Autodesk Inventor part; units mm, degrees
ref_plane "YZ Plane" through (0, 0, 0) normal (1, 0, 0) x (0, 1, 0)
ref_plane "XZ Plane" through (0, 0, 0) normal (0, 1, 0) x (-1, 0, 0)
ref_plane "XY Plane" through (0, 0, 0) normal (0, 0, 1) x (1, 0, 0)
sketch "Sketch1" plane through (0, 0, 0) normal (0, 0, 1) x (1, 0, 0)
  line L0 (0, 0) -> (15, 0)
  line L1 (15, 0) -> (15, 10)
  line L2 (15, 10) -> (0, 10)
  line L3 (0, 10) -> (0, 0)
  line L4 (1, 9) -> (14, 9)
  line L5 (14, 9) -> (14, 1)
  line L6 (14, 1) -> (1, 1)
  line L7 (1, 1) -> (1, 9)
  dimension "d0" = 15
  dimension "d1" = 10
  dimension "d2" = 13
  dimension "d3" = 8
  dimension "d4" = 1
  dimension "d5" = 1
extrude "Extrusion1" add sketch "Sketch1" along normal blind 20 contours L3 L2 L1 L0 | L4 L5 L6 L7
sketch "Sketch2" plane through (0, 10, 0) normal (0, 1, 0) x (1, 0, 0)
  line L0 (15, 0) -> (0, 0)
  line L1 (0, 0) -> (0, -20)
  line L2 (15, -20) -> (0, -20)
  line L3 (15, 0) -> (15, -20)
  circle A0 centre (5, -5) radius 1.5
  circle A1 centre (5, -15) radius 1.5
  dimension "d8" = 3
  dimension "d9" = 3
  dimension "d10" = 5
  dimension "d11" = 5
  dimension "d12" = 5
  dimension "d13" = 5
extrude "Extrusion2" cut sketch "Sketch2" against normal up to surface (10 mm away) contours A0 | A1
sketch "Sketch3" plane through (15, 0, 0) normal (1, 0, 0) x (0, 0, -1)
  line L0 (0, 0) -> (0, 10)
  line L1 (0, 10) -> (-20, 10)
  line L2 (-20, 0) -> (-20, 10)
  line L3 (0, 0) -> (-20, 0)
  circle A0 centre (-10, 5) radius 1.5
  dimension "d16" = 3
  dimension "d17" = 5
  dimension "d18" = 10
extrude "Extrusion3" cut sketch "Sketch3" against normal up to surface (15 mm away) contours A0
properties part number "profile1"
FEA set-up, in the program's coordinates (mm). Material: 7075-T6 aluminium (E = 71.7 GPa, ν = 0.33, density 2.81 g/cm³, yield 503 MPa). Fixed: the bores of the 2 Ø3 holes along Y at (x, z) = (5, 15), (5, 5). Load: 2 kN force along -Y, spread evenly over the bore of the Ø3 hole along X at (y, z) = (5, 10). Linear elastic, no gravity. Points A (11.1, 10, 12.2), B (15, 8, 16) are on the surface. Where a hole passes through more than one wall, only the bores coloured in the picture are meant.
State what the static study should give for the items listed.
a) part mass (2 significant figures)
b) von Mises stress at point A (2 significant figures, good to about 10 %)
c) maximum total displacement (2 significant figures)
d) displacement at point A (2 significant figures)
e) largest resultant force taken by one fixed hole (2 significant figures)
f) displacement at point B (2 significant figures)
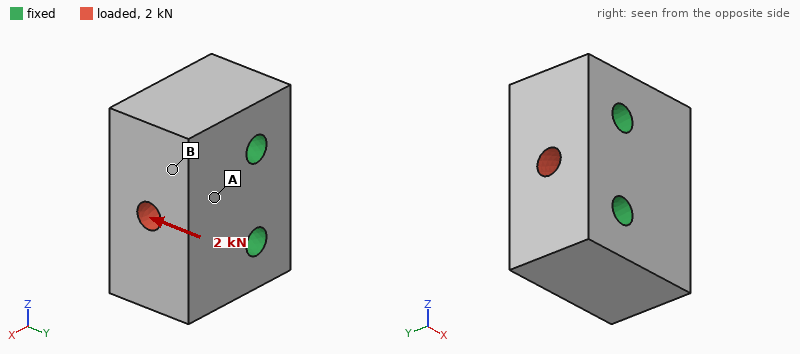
7.7 g
11 MPa
4.4 µm
2.8 µm
1.0 kN
2.7 µm
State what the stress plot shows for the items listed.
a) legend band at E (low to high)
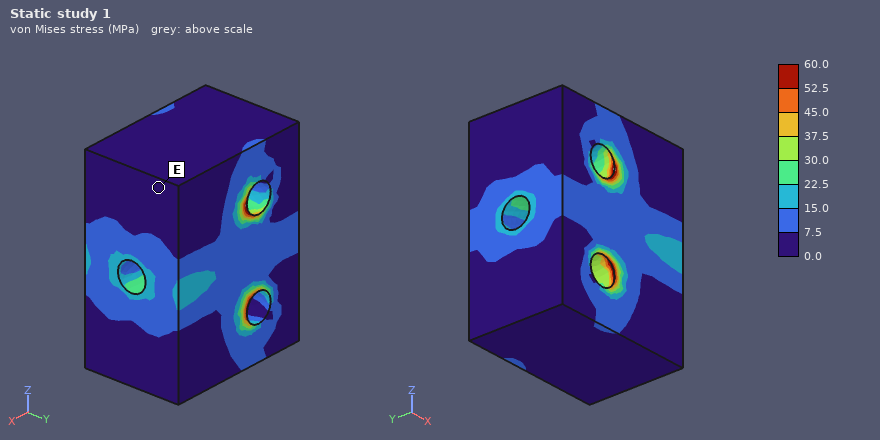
0.0 to 7.5 MPa
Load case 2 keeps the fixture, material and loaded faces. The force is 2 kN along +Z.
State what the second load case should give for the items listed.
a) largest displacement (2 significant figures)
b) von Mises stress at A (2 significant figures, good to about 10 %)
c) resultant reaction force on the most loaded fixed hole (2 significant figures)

2.6 µm
8.5 MPa
1.1 kN
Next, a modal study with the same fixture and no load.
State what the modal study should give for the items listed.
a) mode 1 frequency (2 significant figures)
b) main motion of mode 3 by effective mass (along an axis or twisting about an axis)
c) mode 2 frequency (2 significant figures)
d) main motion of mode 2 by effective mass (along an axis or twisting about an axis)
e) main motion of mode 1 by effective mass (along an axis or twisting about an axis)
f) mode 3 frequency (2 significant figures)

53 kHz
twisting about X
57 kHz
along Z
along Y
66 kHz
